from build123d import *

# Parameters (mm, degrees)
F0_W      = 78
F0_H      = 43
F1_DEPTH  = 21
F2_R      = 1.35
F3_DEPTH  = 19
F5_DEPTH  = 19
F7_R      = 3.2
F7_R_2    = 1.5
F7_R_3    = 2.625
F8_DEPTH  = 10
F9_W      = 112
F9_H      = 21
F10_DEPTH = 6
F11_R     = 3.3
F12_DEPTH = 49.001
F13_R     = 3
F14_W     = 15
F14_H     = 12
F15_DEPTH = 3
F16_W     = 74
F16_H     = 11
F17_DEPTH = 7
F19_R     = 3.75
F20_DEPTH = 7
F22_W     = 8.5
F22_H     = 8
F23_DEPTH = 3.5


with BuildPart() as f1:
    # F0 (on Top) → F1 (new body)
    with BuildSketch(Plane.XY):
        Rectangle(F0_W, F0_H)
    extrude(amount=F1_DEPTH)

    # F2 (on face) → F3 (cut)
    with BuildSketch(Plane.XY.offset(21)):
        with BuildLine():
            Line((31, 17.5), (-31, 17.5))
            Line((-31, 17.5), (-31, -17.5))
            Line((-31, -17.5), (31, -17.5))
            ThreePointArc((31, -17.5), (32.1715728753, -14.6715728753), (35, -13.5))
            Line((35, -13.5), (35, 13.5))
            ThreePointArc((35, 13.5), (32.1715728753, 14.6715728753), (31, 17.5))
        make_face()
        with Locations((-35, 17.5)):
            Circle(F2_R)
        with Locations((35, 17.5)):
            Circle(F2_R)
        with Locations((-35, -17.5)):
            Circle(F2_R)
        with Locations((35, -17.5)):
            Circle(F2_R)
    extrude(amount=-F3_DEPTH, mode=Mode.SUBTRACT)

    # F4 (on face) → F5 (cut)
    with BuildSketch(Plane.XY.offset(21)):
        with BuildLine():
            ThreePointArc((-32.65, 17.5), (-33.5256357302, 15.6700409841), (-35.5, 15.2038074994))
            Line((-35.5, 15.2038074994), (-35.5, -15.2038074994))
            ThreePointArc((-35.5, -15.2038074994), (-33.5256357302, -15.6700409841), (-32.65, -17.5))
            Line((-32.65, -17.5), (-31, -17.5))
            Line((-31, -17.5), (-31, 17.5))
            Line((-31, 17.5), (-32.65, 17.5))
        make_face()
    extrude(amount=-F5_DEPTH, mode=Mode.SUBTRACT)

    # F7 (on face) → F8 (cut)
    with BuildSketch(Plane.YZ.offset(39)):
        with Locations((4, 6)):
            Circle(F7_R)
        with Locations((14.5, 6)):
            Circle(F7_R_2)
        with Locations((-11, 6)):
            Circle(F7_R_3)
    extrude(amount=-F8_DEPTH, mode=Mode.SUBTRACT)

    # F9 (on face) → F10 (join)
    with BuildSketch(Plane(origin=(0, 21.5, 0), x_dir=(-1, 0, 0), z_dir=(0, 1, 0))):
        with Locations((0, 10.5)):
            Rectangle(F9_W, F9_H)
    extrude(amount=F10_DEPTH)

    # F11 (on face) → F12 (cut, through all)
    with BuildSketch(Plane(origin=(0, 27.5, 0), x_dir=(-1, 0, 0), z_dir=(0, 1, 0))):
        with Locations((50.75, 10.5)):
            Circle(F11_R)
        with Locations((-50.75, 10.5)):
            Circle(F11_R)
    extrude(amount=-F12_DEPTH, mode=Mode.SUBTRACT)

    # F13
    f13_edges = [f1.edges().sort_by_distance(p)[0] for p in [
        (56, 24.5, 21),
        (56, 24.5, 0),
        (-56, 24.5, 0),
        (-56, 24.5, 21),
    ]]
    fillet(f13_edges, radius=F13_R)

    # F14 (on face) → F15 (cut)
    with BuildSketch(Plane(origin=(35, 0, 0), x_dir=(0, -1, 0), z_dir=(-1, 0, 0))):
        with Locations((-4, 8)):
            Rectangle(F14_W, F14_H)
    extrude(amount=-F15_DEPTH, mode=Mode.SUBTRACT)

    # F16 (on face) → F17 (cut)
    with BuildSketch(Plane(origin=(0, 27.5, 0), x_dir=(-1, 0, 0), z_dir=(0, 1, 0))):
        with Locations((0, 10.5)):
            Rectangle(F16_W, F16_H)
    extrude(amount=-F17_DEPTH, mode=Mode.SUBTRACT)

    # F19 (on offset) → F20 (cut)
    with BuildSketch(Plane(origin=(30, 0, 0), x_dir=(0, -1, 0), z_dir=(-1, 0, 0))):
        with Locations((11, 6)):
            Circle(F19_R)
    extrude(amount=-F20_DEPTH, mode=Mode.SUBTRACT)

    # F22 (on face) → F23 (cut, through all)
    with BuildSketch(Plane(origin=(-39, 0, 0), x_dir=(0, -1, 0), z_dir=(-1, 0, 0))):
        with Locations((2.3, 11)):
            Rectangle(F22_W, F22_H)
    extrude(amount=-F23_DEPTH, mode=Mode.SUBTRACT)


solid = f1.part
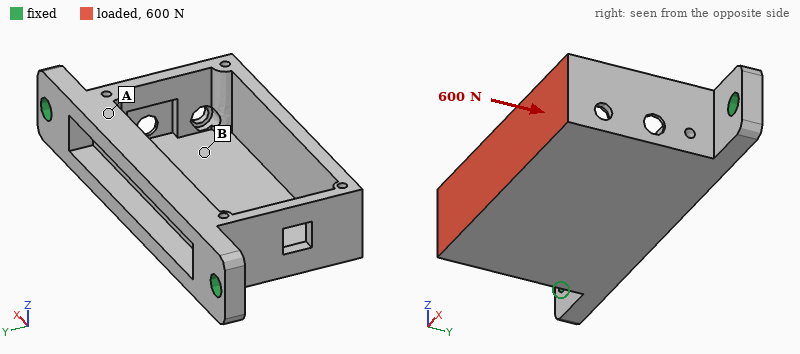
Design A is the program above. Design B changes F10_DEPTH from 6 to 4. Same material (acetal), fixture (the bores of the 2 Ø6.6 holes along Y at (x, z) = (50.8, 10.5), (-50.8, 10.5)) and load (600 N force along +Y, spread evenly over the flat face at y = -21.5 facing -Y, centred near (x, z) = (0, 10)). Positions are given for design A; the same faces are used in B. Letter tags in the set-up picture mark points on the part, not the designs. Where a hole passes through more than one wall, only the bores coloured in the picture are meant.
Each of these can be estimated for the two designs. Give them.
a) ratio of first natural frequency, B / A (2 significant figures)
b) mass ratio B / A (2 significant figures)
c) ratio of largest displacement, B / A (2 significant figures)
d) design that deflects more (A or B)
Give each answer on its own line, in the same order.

0.69
0.90
1.1
B
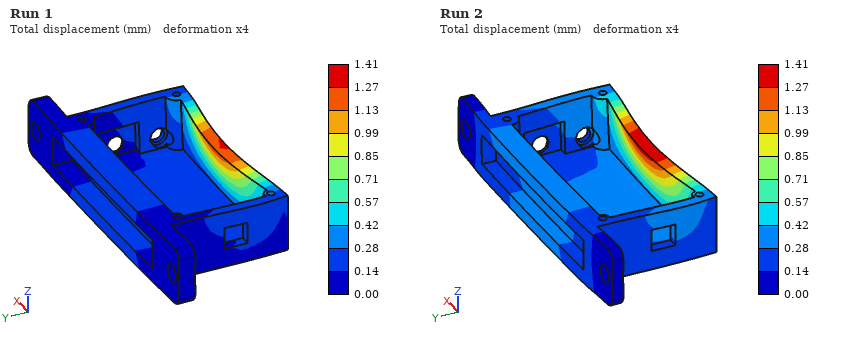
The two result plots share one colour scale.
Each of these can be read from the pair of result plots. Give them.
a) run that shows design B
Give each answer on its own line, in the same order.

Run 2
